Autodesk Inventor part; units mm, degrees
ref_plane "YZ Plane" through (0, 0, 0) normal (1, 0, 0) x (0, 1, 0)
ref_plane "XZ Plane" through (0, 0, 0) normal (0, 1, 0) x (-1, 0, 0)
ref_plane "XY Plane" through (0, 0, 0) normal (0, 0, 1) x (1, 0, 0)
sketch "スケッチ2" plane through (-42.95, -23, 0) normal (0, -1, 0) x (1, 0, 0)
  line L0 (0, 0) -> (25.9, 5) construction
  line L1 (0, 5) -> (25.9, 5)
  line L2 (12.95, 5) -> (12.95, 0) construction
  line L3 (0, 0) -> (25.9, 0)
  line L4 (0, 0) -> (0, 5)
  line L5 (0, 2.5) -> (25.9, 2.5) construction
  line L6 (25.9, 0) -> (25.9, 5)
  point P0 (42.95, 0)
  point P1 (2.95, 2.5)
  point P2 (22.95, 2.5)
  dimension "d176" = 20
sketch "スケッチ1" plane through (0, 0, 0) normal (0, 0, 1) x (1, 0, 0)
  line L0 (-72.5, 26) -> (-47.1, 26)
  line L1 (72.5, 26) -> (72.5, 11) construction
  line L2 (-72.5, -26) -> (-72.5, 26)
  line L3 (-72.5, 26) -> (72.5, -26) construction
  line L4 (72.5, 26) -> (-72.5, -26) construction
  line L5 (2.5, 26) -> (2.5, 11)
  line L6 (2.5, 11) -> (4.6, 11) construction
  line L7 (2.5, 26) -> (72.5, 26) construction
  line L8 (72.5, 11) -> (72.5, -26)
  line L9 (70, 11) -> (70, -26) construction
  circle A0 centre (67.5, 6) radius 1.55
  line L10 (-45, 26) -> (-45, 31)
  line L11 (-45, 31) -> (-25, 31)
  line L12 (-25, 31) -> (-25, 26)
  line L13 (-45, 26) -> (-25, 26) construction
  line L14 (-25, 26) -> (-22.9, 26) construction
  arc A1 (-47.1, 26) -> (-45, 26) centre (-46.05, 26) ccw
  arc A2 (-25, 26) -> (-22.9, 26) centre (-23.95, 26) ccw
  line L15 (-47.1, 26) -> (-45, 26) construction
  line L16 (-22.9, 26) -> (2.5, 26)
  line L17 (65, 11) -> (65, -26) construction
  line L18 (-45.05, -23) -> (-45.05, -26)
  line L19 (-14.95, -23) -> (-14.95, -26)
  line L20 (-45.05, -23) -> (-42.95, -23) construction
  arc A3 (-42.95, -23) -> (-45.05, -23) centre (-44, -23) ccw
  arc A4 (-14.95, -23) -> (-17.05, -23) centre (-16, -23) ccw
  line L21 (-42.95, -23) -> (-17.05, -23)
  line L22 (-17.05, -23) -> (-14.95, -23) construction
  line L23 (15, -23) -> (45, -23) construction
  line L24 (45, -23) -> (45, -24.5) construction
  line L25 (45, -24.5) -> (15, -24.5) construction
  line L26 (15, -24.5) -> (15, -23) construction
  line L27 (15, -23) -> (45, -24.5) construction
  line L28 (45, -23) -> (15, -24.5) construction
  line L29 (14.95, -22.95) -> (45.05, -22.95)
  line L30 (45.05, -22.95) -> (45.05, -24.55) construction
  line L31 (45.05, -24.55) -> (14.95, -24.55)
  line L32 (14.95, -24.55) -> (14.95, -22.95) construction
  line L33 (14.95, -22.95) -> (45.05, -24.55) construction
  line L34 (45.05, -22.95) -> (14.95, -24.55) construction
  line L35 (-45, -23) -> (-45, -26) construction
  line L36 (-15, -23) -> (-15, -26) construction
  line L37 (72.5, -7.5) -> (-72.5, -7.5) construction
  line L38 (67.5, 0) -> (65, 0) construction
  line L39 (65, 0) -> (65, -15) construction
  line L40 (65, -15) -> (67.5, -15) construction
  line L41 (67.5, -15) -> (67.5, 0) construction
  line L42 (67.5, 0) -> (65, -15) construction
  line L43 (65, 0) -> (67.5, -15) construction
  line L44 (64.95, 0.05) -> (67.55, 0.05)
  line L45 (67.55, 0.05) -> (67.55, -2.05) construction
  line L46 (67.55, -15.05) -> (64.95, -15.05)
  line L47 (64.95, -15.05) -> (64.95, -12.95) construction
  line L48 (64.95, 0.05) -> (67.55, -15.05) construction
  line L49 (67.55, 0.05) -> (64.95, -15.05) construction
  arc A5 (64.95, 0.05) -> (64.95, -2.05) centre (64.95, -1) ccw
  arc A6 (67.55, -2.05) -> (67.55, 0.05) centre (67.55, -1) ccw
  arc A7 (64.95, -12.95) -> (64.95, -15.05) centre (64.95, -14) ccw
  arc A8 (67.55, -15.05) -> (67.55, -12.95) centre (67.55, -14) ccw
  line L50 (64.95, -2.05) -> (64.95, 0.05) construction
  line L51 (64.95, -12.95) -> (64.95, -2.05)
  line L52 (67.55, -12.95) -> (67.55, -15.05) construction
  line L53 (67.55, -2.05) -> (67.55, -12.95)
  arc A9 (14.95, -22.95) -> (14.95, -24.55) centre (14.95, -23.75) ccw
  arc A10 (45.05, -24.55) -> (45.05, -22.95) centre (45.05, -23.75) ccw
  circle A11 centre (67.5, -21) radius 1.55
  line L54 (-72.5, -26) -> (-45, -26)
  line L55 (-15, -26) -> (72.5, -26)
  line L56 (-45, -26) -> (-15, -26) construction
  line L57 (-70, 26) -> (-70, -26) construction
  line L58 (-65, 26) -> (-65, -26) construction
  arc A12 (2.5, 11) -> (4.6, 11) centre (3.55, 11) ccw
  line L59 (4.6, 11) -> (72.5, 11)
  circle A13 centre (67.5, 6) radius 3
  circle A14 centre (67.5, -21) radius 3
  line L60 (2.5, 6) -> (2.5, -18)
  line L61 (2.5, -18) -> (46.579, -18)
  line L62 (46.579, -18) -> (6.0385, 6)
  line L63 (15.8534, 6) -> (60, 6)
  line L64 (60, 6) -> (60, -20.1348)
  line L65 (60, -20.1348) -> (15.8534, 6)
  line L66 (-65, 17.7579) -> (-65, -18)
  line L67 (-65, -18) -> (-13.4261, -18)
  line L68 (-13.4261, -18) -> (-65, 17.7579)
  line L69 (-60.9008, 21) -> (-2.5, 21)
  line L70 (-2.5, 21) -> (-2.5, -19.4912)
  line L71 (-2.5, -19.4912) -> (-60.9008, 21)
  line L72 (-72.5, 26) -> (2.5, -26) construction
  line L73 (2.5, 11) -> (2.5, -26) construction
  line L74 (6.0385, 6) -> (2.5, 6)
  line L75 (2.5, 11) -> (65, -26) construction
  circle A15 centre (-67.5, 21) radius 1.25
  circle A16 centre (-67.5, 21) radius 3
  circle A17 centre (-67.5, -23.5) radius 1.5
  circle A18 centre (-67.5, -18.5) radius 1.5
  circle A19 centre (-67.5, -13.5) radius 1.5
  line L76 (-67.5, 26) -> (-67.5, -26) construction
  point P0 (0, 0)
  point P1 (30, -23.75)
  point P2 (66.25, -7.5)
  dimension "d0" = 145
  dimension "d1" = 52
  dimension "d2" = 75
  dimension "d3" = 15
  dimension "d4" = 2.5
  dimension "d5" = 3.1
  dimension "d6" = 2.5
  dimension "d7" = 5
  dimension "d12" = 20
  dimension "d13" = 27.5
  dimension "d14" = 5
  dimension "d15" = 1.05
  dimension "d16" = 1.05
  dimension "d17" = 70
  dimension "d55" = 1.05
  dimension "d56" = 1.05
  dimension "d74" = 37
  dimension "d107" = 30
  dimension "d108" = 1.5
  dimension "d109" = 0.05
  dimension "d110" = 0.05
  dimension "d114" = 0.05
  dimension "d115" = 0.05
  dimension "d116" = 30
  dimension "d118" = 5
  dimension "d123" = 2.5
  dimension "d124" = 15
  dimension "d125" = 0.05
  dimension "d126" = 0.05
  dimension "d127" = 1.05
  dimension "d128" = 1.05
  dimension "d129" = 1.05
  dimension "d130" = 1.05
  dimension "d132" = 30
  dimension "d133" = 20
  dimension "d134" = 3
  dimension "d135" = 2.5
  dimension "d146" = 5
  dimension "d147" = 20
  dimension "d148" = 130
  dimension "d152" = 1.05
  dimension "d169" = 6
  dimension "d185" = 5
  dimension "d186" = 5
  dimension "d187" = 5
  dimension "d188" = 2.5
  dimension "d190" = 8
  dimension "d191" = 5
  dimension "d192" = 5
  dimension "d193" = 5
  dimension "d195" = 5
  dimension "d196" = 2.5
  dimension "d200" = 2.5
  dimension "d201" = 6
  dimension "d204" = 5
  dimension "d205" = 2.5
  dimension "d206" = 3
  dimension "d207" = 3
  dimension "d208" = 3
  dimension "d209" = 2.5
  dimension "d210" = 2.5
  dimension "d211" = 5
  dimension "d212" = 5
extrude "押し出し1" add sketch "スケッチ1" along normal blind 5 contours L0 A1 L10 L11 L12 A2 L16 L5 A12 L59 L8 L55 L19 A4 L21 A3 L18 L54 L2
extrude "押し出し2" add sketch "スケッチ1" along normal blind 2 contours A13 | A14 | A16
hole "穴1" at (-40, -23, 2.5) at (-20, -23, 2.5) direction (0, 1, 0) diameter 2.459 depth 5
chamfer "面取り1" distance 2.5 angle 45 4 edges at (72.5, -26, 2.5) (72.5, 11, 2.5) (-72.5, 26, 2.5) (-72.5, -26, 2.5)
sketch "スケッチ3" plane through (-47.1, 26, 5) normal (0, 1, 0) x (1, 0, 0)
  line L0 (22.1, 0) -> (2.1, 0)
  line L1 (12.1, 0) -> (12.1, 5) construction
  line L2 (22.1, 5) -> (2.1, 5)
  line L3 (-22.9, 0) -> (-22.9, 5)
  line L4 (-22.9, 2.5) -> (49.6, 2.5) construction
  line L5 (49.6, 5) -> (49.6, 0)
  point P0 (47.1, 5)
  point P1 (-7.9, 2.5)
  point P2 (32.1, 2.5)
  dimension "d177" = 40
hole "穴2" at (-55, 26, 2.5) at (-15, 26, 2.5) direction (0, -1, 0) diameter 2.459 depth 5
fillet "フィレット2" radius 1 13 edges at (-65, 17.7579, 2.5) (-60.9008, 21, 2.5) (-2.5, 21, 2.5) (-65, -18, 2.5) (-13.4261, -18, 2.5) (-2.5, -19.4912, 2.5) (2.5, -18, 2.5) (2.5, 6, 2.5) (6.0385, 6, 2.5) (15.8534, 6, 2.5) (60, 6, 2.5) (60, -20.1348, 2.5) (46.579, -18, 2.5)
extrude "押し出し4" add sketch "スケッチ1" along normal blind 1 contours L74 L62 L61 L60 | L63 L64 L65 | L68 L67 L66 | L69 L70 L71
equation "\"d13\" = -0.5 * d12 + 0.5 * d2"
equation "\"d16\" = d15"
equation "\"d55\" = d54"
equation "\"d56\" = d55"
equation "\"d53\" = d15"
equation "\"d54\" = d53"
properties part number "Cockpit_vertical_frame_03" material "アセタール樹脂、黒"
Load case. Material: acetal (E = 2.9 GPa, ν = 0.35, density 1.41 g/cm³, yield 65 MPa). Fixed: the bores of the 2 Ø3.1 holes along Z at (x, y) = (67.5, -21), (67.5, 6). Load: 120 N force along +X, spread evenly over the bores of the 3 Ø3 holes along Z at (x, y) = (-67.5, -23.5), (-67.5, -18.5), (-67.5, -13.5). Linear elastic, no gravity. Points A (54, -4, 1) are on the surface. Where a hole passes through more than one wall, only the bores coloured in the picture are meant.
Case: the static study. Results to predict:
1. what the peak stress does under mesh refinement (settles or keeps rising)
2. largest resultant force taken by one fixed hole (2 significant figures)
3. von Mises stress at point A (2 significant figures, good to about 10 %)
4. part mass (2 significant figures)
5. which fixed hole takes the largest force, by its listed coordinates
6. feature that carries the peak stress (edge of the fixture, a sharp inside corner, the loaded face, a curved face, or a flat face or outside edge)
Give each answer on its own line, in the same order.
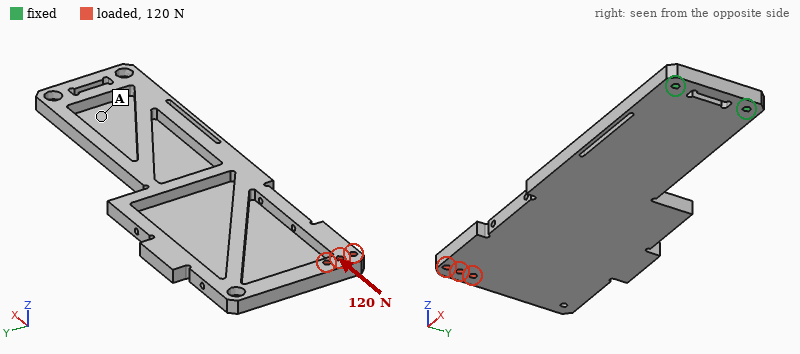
keeps rising
110 N
1.0 MPa
26 g
(67.5, -21)
edge of the fixture
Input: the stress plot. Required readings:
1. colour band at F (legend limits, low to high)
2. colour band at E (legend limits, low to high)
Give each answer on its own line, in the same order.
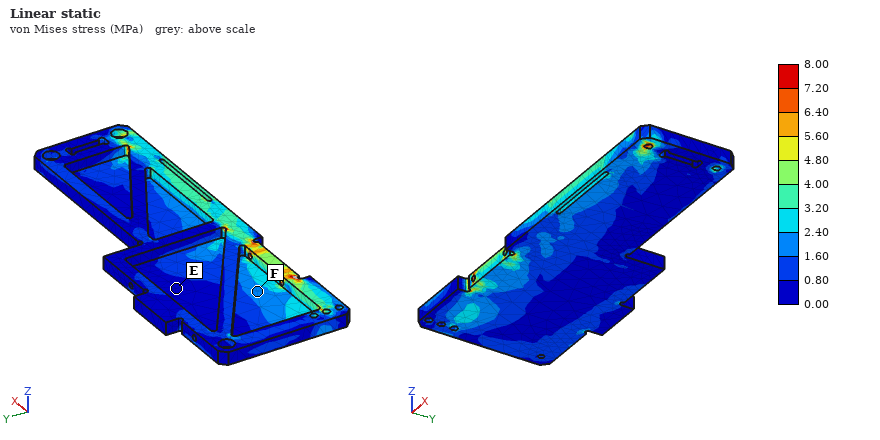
1.60 to 2.40 MPa
0.00 to 0.80 MPa
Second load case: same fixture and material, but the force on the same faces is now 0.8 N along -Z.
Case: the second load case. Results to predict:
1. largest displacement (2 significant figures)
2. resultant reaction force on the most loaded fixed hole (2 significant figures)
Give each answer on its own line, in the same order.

1.5 mm
3.1 N
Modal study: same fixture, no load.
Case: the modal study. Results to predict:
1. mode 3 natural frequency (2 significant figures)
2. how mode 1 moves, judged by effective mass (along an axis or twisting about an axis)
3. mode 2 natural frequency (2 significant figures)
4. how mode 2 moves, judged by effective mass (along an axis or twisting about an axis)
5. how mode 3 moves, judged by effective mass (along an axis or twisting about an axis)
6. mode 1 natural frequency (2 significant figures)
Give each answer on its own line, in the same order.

270 Hz
along Z
180 Hz
twisting about X
along Z
43 Hz
